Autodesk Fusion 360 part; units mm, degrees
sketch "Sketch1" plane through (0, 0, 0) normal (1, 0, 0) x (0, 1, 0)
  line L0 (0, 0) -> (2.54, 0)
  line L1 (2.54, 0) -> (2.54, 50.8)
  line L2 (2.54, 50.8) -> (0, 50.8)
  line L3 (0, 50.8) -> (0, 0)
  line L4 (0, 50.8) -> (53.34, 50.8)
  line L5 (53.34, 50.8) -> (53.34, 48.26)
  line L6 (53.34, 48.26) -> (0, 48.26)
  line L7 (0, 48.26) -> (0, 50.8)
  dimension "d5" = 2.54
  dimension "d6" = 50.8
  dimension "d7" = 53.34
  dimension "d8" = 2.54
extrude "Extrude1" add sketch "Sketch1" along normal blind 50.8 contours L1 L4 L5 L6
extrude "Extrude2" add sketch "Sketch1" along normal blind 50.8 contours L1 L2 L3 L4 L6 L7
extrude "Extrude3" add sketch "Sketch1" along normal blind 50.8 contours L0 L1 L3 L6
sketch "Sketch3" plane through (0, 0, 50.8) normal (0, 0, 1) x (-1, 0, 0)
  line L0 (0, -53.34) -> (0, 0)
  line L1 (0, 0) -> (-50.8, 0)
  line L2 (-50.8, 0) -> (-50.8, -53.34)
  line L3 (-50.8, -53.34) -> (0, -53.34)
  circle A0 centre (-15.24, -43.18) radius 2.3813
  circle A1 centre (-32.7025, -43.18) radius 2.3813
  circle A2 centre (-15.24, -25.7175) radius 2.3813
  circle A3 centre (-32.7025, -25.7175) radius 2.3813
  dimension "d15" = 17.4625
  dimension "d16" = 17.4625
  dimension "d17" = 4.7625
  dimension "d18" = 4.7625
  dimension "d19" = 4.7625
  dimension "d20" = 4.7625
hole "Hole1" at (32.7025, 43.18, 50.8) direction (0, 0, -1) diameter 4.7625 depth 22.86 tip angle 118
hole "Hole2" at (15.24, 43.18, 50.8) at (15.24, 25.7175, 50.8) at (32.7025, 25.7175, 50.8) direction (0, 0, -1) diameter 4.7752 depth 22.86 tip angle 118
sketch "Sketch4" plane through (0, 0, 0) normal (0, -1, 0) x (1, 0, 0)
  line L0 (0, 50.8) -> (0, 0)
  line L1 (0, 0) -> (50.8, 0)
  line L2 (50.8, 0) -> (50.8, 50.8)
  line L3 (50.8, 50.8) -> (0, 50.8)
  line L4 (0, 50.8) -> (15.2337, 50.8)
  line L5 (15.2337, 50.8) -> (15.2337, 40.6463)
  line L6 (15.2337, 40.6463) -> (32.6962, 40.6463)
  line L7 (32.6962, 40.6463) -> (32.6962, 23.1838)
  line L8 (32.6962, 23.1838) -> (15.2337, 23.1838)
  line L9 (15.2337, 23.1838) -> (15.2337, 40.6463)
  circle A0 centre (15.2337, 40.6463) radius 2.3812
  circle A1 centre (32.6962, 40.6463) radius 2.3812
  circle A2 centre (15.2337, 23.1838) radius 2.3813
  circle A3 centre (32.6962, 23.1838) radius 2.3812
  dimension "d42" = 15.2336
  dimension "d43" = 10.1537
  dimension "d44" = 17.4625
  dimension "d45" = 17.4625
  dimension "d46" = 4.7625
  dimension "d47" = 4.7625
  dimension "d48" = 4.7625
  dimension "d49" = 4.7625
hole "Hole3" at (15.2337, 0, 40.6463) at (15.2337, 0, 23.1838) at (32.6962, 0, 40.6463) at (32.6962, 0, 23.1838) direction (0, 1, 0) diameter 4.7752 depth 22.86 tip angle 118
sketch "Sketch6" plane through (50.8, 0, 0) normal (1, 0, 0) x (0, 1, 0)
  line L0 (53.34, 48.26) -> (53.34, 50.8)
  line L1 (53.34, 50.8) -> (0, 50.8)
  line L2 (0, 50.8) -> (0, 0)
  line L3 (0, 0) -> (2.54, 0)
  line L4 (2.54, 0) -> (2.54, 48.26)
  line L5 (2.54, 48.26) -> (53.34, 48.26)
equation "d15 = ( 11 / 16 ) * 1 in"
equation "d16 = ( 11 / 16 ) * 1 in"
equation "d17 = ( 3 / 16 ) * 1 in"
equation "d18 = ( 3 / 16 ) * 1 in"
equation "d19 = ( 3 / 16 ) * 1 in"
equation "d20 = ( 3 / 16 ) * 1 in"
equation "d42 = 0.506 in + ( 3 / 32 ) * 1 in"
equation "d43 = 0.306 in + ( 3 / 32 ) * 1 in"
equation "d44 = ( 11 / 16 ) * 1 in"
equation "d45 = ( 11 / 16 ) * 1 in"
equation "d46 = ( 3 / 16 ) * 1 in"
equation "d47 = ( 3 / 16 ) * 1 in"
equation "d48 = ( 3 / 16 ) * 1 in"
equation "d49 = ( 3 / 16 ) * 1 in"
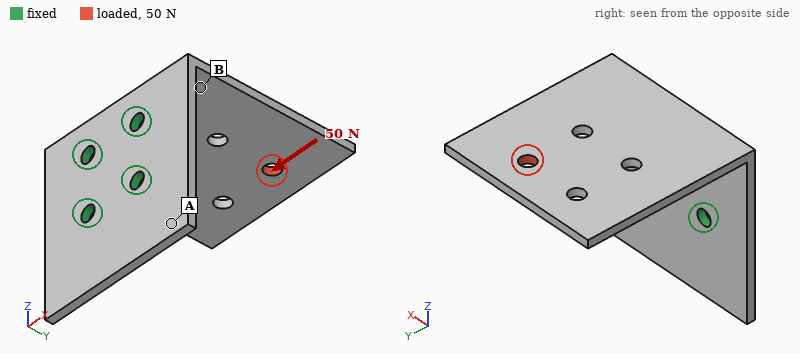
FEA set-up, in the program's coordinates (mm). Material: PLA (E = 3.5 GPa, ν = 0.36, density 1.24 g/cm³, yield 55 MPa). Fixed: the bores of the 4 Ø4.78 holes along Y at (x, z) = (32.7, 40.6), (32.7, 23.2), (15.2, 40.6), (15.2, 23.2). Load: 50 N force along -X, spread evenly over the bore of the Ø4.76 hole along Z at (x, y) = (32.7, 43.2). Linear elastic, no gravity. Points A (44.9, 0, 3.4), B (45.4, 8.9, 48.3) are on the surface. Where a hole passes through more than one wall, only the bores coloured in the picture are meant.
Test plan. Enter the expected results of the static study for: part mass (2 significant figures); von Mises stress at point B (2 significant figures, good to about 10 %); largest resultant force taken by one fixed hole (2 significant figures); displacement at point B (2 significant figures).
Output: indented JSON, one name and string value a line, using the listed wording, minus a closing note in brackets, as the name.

{
  "part mass": "16 g",
  "von Mises stress at point B": "4.4 MPa",
  "largest resultant force taken by one fixed hole": "100 N",
  "displacement at point B": "0.26 mm"
}
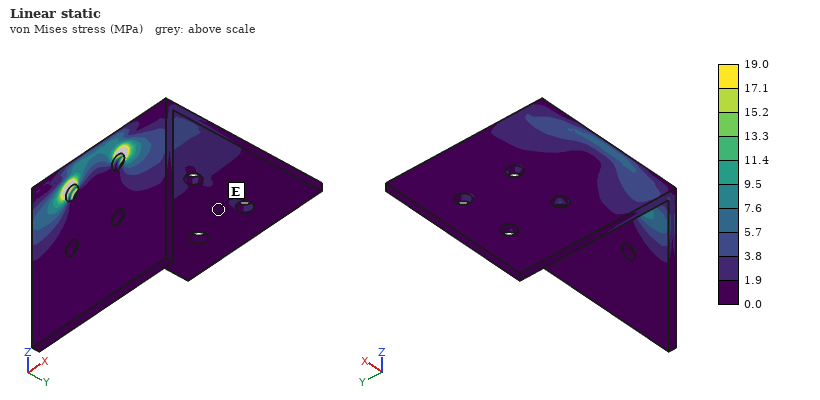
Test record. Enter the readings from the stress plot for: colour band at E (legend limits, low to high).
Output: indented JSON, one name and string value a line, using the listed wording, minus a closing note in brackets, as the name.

{
  "colour band at E": "0.0 to 1.9 MPa"
}
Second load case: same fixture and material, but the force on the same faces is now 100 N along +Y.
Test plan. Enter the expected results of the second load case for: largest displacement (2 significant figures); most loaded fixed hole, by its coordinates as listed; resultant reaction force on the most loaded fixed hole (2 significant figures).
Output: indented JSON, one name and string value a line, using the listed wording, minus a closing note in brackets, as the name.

{
  "largest displacement": "0.93 mm",
  "most loaded fixed hole, by its coordinates as listed": "(32.7, 40.6)",
  "resultant reaction force on the most loaded fixed hole": "96 N"
}
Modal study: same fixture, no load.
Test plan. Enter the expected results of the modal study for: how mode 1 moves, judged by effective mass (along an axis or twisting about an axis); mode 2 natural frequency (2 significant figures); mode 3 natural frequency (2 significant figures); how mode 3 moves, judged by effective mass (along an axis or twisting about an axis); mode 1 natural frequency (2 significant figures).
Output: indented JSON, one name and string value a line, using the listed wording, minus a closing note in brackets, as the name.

{
  "how mode 1 moves, judged by effective mass": "along Z",
  "mode 2 natural frequency": "540 Hz",
  "mode 3 natural frequency": "780 Hz",
  "how mode 3 moves, judged by effective mass": "along X",
  "mode 1 natural frequency": "210 Hz"
}
